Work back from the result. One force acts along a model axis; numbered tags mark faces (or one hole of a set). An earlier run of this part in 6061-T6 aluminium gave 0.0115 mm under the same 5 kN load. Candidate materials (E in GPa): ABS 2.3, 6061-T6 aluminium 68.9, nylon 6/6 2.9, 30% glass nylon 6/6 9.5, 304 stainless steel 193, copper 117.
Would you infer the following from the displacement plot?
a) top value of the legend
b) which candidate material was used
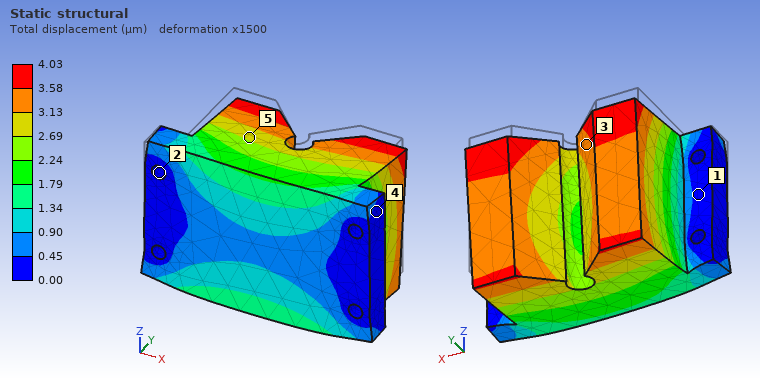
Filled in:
4.03 µm
304 stainless steel
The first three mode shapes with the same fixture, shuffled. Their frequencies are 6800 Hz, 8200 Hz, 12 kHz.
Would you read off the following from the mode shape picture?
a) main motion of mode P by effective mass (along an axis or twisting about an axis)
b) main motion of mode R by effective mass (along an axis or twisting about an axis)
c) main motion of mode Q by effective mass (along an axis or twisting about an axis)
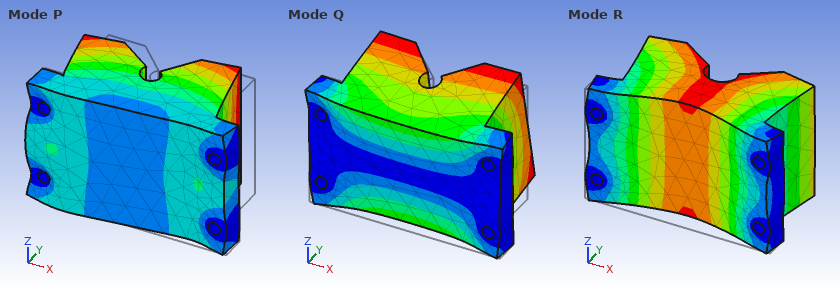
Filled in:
along X
along Y
along Z
